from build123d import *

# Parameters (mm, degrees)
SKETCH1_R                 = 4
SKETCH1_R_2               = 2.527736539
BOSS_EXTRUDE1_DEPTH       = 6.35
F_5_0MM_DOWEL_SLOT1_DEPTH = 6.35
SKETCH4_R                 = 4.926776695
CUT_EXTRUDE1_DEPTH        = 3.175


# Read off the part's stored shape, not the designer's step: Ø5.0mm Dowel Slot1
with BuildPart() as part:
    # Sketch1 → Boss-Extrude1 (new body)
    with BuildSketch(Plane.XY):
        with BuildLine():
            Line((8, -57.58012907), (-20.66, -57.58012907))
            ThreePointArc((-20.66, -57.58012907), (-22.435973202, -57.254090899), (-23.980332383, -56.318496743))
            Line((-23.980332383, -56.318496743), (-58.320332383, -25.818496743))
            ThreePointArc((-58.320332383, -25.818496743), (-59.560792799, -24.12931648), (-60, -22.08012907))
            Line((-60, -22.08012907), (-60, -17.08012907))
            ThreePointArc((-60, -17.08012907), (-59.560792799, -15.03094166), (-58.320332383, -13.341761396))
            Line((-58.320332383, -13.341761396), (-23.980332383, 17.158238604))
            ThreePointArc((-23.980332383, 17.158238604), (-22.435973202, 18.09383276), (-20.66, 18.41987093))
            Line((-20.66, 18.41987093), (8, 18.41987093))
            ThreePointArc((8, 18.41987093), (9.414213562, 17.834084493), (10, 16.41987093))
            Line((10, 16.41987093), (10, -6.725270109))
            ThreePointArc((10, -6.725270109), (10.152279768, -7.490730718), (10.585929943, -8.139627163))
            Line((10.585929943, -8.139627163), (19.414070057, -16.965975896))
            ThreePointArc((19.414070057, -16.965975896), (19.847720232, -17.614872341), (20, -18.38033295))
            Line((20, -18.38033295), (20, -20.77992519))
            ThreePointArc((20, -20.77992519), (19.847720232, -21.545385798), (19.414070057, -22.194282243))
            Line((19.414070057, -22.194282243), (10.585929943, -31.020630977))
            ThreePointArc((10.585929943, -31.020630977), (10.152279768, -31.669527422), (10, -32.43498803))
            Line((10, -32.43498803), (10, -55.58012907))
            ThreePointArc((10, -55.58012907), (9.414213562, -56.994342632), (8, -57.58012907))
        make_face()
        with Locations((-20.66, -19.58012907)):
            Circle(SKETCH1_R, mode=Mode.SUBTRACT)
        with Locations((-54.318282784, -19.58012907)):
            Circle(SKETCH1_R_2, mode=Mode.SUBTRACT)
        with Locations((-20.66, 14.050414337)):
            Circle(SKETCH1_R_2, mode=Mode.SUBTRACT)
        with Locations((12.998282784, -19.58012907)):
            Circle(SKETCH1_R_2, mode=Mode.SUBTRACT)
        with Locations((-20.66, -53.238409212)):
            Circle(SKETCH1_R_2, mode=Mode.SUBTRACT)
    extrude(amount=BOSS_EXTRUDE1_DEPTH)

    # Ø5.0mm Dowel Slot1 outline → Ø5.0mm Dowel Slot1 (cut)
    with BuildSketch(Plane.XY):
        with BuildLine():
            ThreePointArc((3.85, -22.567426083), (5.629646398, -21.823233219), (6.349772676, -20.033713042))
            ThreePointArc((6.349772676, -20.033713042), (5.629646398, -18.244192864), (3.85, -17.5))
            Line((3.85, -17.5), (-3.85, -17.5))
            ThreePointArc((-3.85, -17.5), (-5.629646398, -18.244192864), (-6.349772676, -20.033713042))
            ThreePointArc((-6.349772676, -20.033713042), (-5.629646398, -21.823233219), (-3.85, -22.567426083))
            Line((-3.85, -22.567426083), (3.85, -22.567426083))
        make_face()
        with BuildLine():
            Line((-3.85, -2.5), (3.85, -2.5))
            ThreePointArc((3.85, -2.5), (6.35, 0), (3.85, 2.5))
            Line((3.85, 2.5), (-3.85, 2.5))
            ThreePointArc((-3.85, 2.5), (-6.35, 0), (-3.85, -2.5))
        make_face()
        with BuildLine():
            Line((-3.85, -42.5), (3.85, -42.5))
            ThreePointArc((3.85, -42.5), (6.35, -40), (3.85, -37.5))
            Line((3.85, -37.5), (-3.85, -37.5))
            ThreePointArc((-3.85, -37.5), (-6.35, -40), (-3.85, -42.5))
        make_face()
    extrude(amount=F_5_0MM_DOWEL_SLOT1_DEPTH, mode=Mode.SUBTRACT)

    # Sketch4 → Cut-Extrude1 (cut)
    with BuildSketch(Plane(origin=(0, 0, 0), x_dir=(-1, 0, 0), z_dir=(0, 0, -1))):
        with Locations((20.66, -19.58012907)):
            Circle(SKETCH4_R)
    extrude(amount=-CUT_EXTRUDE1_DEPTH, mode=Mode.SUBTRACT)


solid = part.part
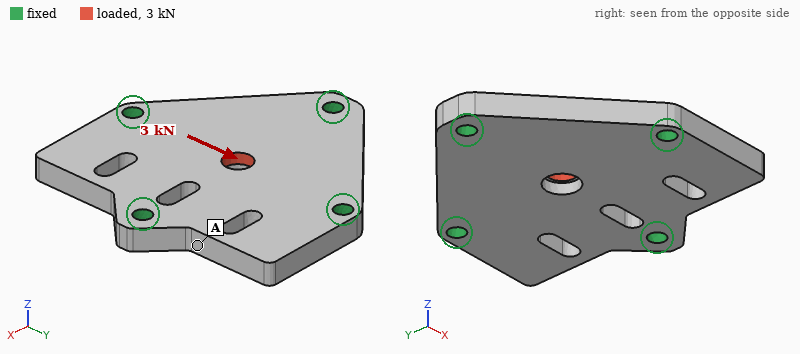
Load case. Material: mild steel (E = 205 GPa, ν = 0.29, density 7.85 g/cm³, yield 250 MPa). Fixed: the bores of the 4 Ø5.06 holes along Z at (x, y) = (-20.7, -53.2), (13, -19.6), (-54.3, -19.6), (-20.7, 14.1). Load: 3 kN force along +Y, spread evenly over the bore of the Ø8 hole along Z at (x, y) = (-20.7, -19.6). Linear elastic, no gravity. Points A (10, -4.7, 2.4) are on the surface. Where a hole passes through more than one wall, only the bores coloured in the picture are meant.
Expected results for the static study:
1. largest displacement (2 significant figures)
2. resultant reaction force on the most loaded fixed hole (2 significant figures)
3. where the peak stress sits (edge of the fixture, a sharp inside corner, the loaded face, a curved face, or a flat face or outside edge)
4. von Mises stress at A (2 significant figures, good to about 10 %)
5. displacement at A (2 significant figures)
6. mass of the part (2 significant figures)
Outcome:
2.5 µm
1.1 kN
a sharp inside corner
7.7 MPa
0.56 µm
190 g
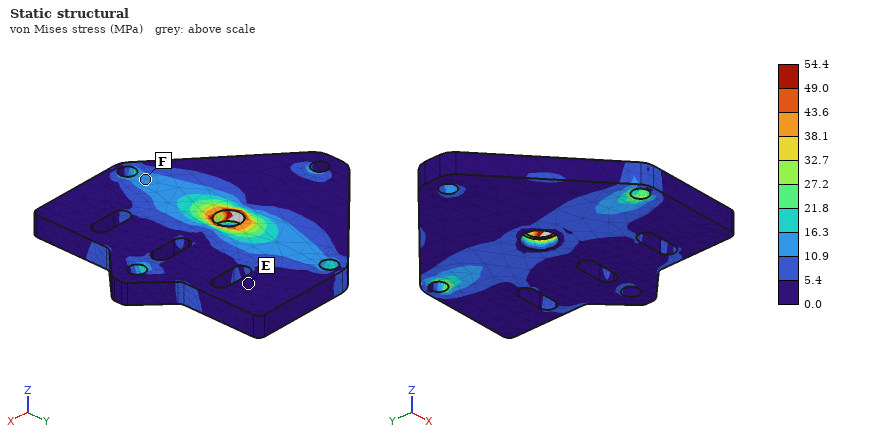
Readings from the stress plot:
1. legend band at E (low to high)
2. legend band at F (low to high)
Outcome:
0.0 to 5.4 MPa
10.9 to 16.3 MPa
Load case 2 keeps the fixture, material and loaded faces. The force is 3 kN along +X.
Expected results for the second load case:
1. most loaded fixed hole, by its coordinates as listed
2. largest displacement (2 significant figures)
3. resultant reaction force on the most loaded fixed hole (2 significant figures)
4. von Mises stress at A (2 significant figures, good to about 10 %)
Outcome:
(-54.3, -19.6)
2.9 µm
1.2 kN
10 MPa
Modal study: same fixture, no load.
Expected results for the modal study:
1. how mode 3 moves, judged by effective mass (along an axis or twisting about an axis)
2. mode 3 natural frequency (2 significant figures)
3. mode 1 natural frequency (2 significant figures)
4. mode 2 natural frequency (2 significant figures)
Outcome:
along Z
9500 Hz
8600 Hz
8700 Hz
